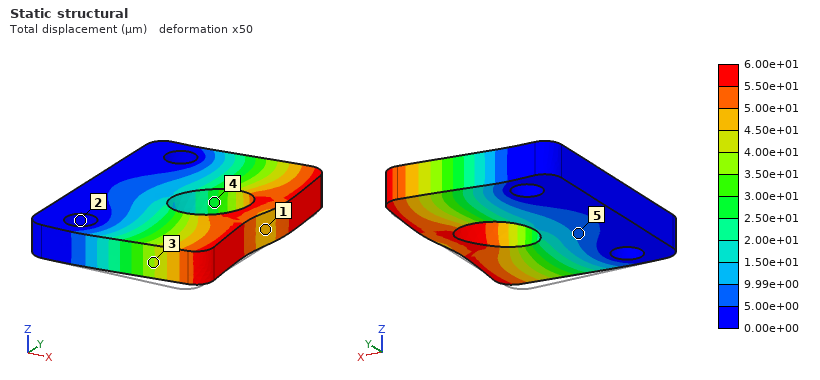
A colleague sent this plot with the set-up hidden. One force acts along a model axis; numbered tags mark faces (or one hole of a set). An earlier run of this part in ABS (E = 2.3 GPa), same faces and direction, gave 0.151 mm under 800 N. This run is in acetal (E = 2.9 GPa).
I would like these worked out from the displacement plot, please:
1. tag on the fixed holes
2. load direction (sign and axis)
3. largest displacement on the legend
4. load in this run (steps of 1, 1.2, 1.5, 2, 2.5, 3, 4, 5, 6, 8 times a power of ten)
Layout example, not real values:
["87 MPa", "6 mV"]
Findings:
["2", "+Y", "6.00e+01 µm", "400 N"]
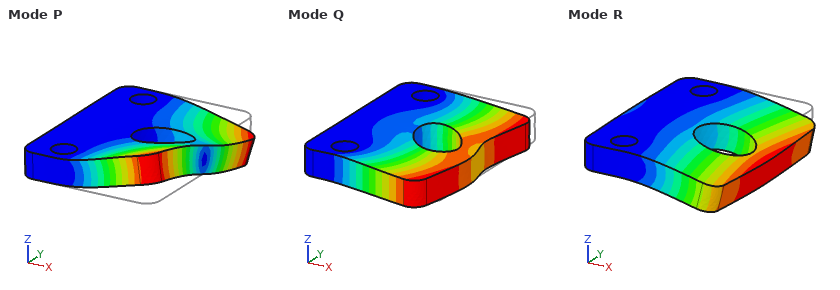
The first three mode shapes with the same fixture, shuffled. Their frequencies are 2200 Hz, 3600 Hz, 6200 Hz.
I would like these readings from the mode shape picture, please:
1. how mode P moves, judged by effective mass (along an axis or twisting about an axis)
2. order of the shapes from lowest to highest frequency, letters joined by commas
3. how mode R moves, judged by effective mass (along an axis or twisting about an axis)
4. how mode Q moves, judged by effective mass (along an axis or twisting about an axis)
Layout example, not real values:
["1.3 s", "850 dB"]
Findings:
["twisting about X", "R, P, Q", "along Z", "along Y"]
